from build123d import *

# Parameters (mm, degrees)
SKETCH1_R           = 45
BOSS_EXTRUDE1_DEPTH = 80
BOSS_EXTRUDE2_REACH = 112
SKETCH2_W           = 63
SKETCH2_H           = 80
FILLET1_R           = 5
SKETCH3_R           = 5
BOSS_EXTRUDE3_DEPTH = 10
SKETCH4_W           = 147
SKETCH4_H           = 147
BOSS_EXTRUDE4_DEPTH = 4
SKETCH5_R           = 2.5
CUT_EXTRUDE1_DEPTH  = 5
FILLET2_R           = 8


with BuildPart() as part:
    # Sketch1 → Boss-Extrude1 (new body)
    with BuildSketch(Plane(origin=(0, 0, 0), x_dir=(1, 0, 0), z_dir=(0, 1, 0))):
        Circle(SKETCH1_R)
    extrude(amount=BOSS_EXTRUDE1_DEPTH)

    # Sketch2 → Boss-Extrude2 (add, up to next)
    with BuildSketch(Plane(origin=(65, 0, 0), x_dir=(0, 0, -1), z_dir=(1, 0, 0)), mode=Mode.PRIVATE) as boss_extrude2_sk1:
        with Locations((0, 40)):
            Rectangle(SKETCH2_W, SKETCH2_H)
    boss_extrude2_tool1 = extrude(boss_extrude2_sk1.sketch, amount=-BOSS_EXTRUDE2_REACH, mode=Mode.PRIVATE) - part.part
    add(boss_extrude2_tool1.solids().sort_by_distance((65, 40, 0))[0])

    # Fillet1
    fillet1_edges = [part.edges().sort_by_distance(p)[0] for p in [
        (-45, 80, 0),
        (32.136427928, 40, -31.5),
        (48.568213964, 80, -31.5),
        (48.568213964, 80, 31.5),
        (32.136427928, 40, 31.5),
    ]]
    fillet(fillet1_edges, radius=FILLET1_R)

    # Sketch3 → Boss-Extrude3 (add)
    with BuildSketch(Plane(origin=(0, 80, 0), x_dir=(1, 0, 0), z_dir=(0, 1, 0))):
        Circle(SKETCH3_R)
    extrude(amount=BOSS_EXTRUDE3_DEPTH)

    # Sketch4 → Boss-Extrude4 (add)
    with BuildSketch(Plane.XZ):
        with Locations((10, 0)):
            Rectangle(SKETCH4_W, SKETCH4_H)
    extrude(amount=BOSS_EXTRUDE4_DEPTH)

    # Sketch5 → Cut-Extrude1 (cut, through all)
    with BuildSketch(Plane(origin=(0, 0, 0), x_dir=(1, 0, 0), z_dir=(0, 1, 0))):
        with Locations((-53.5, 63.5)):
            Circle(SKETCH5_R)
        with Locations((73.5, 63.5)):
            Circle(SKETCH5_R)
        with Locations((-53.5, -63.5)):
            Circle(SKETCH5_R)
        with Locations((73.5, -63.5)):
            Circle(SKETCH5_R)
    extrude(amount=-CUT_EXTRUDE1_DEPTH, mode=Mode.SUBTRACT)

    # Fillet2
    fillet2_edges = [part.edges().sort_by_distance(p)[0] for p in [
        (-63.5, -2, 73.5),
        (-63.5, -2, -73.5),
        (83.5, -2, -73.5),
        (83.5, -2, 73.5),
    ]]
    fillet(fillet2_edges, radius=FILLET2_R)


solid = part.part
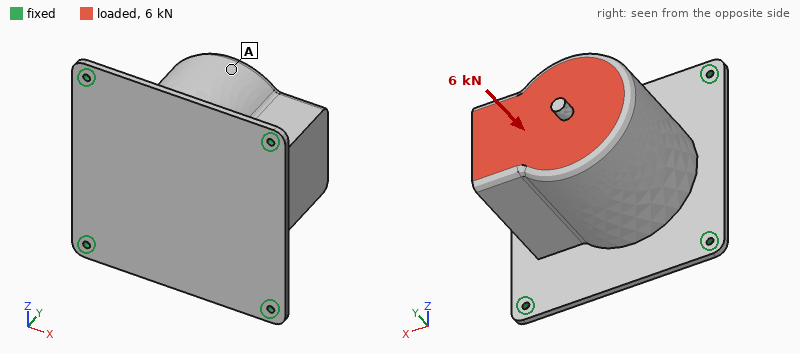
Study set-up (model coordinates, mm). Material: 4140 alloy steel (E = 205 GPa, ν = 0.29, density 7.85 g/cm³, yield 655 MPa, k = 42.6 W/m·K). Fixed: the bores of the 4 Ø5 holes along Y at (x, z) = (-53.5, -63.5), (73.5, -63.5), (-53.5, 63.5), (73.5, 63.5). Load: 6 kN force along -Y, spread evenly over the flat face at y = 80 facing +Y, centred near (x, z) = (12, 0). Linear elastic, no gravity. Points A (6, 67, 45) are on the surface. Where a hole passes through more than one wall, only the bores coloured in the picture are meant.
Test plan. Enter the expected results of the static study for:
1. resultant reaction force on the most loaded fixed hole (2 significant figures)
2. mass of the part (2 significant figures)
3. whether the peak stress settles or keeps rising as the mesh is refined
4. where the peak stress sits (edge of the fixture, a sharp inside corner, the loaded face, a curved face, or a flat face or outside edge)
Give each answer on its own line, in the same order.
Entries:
1.7 kN
5.6 kg
keeps rising
edge of the fixture
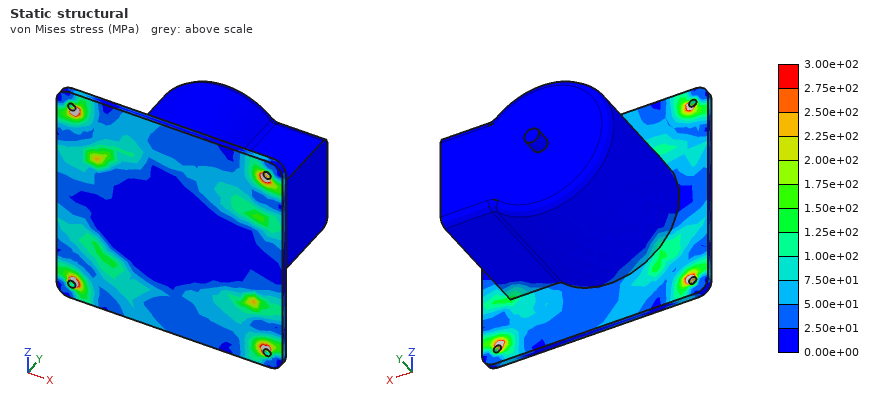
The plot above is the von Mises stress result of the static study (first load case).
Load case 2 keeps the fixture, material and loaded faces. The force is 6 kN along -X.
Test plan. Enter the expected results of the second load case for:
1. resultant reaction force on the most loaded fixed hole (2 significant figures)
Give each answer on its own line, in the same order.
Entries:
2.9 kN
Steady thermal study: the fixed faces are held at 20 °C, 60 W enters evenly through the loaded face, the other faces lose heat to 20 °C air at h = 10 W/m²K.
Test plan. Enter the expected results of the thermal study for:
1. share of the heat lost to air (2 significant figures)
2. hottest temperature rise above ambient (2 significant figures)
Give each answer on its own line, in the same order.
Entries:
49 %
63 K
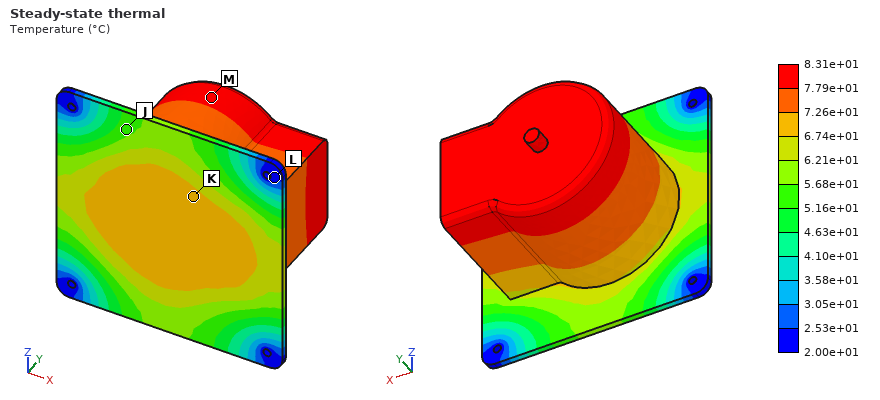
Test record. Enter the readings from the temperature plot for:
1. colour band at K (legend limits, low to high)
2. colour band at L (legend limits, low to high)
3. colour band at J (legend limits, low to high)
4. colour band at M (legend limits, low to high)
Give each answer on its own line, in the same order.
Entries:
6.74e+01 to 7.26e+01 °C
2.00e+01 to 2.53e+01 °C
5.16e+01 to 5.68e+01 °C
7.79e+01 to 8.31e+01 °C
